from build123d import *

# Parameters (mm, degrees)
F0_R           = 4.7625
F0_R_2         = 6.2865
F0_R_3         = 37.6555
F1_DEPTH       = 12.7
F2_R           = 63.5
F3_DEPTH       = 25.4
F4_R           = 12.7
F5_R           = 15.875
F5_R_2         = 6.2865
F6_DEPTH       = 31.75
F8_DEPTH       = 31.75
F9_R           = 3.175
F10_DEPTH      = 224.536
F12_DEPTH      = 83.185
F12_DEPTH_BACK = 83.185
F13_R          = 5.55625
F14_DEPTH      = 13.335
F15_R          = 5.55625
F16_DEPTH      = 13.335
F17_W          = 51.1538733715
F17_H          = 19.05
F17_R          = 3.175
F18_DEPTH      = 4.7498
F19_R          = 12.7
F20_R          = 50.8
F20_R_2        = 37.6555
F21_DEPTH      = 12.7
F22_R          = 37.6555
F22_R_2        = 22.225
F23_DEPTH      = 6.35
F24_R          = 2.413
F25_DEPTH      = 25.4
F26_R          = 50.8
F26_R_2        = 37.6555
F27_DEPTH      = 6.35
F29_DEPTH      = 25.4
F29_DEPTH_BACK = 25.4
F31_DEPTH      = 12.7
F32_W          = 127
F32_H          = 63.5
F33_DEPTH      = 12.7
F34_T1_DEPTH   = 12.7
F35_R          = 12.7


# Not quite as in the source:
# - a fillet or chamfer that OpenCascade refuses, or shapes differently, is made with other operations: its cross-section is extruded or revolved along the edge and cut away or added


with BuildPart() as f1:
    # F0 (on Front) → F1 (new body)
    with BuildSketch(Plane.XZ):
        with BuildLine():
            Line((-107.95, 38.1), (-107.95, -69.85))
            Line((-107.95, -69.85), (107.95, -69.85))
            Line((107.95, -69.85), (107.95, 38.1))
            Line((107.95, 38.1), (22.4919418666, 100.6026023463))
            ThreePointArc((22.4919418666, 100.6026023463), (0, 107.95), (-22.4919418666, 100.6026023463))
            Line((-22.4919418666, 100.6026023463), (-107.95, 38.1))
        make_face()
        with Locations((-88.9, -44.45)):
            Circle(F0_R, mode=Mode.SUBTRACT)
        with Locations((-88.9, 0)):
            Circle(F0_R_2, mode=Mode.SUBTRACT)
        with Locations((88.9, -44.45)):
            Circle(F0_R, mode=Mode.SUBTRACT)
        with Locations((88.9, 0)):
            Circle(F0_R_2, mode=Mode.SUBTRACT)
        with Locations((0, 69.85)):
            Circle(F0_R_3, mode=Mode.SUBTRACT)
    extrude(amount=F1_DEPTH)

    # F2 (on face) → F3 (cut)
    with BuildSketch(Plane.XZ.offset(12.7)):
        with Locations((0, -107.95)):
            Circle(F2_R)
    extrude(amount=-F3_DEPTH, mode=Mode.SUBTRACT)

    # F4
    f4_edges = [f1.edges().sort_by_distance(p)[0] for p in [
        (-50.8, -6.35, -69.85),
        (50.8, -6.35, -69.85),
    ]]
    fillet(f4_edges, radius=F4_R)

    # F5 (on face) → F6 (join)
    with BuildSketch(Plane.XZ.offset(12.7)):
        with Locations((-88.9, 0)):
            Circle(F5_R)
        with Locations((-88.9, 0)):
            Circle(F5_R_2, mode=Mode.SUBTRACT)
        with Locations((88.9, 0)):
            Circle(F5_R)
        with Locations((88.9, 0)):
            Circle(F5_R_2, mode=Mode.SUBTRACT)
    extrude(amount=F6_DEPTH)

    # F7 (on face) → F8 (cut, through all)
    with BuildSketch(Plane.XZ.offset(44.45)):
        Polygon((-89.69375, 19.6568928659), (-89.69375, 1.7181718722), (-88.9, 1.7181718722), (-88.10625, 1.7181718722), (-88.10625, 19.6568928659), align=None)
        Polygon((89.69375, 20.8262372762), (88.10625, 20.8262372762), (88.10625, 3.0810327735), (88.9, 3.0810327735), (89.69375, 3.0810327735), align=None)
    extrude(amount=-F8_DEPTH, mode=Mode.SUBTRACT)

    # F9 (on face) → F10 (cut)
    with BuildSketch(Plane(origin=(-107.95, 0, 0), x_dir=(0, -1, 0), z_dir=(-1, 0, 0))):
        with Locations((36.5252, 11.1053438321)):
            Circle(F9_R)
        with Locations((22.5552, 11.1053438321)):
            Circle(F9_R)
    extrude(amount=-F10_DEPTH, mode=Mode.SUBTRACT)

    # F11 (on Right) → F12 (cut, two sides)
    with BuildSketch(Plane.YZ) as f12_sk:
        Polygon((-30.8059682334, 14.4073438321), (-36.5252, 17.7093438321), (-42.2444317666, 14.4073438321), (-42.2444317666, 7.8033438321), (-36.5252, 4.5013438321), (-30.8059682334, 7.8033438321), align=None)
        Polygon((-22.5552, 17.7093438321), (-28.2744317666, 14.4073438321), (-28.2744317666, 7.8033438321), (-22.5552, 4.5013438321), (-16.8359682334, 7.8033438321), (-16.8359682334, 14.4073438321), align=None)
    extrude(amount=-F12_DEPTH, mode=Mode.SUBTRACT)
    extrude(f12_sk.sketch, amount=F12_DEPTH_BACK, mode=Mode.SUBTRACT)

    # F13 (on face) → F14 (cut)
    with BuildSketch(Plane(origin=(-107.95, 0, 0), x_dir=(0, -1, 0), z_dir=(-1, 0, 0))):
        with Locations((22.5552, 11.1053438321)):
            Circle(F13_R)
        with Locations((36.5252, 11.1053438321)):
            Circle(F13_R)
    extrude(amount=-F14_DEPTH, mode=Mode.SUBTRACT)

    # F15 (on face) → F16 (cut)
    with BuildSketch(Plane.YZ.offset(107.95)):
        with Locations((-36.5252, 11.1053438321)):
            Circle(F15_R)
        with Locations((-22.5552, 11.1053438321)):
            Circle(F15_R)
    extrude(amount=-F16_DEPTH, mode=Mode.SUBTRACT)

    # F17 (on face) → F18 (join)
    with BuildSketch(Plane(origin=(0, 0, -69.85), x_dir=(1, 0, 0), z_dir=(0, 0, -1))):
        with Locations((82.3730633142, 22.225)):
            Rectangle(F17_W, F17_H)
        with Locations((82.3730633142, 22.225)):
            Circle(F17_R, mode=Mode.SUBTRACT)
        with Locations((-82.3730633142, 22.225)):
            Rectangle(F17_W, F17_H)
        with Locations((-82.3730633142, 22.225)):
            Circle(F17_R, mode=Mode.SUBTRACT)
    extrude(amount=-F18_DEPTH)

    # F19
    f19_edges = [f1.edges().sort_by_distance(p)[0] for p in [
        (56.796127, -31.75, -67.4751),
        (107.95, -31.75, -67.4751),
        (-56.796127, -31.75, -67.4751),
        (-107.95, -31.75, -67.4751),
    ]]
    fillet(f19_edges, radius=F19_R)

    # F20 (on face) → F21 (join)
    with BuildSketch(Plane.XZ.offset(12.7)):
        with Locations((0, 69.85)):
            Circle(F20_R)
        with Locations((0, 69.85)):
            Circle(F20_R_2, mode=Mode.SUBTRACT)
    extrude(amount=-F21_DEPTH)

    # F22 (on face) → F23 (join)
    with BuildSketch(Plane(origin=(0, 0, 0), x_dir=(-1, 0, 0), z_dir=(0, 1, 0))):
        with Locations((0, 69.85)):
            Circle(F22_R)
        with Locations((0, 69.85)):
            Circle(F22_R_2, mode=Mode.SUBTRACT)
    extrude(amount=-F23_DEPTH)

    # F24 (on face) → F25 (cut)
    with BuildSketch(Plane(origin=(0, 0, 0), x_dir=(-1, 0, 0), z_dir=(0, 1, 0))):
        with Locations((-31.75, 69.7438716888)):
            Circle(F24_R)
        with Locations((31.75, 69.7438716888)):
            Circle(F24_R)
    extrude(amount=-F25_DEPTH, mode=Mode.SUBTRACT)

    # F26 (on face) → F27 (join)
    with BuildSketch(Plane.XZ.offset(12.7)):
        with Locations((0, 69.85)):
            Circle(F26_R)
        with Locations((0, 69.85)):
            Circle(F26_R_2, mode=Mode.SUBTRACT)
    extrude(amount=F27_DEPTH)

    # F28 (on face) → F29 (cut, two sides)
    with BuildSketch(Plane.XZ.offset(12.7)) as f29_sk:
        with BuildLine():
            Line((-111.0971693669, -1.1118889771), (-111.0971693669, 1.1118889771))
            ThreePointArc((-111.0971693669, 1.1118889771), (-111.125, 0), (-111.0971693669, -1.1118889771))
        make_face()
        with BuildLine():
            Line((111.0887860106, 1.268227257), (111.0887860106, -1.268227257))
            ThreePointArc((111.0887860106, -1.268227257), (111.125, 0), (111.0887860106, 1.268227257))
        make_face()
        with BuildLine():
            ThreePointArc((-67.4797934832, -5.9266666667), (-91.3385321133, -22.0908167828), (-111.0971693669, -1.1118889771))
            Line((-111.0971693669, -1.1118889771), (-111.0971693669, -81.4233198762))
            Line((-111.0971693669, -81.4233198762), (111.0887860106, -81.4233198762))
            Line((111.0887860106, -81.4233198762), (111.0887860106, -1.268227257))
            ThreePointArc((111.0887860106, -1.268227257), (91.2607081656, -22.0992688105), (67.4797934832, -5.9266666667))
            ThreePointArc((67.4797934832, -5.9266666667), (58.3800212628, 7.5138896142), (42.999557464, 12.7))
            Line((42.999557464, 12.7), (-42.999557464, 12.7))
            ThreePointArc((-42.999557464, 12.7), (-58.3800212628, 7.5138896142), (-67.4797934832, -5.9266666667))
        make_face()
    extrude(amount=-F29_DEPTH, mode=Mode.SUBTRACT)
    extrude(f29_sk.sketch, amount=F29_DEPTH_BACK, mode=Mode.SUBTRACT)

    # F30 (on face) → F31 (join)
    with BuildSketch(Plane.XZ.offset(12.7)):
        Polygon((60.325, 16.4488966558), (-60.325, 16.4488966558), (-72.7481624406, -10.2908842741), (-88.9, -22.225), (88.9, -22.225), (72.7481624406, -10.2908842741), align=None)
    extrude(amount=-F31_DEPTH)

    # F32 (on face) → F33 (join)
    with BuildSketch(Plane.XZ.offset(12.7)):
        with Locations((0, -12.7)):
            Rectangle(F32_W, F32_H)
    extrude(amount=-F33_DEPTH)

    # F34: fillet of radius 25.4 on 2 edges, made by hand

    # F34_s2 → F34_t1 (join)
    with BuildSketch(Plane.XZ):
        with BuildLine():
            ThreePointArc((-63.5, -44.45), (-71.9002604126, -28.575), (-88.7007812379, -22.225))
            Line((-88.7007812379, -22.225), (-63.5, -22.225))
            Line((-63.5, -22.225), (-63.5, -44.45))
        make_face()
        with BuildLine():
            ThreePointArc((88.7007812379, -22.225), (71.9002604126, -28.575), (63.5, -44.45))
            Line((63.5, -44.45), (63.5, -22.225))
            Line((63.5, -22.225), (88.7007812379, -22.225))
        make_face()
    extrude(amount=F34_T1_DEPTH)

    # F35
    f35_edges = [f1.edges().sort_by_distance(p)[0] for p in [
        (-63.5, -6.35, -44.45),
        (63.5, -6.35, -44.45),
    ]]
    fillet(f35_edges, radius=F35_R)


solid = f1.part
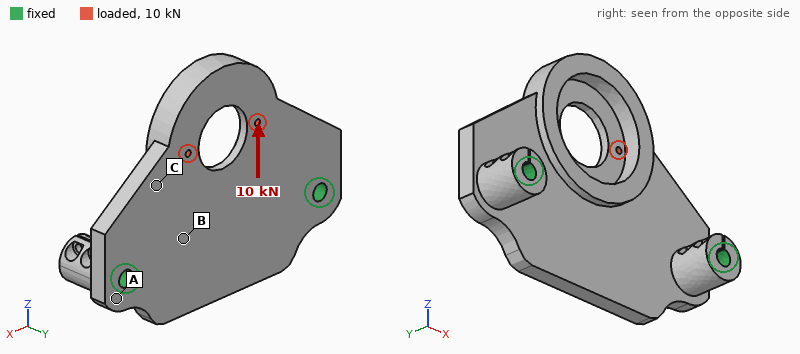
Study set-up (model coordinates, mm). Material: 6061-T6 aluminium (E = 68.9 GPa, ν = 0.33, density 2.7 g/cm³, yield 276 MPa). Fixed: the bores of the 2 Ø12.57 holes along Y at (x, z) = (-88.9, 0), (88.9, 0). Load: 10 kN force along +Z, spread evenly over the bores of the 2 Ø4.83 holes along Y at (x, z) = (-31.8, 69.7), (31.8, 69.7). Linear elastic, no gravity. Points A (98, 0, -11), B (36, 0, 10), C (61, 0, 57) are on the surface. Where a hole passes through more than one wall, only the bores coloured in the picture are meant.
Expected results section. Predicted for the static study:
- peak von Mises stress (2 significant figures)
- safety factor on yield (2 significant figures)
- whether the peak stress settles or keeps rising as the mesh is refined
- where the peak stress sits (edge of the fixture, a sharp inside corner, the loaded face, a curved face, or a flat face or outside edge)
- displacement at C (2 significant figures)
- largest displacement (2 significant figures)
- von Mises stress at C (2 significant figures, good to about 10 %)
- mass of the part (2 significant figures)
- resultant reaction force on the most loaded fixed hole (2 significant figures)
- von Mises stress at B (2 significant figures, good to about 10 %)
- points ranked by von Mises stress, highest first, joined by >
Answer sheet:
94 MPa
2.9
settles
the loaded face
0.036 mm
0.14 mm
14 MPa
930 g
5.2 kN
8.3 MPa
C > B > A
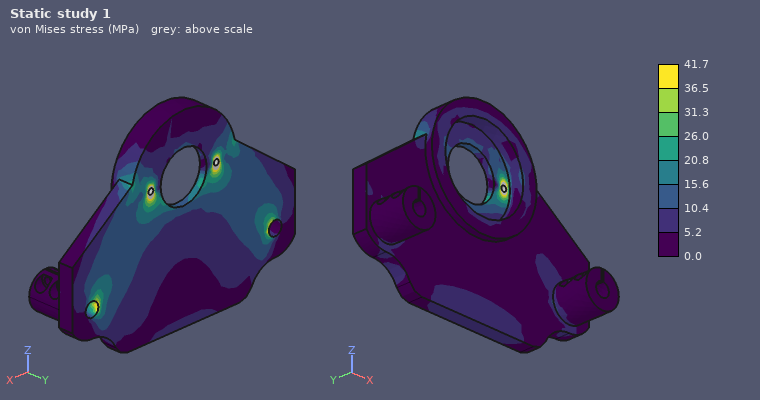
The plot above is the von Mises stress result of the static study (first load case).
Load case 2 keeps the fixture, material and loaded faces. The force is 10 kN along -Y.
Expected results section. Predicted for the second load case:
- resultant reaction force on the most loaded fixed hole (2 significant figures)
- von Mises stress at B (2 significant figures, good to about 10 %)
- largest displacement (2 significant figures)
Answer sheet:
5.0 kN
70 MPa
1.8 mm
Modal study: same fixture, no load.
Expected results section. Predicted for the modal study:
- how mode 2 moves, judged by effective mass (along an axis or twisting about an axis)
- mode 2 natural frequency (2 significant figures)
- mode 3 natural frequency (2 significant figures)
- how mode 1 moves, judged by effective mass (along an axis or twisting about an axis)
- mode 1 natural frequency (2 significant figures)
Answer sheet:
along Y
2100 Hz
2600 Hz
along Y
880 Hz
